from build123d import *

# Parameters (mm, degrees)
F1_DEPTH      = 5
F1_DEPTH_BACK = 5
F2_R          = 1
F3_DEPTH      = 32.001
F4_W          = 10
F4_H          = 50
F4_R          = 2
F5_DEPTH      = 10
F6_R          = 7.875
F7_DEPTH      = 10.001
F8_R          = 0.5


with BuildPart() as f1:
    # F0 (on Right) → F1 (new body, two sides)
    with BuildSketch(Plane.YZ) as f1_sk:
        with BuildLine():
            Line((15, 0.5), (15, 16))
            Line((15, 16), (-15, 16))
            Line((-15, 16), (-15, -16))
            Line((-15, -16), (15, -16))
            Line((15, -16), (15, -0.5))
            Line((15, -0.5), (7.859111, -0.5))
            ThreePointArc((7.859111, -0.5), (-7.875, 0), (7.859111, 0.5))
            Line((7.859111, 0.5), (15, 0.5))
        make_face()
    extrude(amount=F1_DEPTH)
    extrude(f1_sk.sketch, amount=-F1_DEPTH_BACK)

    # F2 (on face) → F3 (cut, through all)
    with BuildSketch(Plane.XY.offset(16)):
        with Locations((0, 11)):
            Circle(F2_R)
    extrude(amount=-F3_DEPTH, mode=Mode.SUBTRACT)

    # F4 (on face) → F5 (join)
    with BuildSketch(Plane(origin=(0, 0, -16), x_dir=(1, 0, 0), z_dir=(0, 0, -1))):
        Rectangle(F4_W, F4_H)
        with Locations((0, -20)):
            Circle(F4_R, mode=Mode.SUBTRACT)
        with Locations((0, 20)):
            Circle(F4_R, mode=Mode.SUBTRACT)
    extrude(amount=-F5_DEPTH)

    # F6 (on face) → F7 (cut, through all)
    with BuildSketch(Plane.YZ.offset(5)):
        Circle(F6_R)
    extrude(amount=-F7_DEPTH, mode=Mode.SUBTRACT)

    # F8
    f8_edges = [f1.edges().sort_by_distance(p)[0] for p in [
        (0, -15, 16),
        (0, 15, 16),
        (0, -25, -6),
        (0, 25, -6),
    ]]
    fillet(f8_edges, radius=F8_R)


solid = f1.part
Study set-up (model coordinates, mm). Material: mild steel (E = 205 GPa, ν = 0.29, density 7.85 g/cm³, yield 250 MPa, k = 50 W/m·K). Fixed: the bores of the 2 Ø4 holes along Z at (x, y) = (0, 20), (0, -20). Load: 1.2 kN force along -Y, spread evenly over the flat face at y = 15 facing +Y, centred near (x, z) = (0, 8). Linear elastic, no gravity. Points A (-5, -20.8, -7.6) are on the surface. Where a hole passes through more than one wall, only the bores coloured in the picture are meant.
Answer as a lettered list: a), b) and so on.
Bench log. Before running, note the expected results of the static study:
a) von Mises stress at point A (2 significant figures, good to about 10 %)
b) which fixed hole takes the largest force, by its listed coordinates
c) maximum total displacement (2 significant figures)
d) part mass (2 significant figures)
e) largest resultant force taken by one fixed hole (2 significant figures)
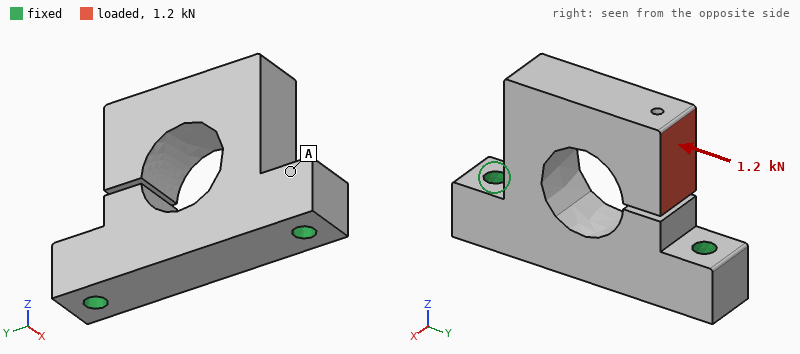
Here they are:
a) 19 MPa
b) (0, -20)
c) 71 µm
d) 73 g
e) 1.2 kN
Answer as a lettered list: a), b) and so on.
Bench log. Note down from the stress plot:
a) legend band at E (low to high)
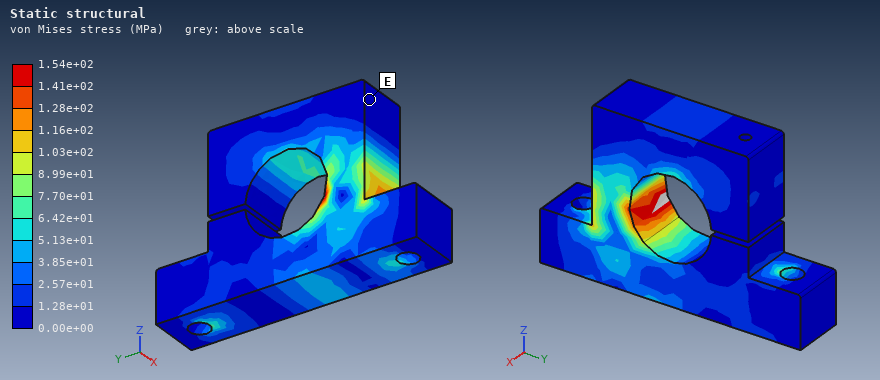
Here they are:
a) 0.00e+00 to 1.28e+01 MPa
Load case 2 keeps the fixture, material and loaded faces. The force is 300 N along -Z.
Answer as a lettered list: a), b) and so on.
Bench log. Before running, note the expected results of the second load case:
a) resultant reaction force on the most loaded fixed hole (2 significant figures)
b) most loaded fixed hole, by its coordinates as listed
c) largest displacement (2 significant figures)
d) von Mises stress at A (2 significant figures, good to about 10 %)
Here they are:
a) 260 N
b) (0, 20)
c) 67 µm
d) 6.2 MPa
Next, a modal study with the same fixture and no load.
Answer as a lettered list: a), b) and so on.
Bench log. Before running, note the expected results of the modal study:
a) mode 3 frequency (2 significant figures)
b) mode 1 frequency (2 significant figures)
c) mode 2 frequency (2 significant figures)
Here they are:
a) 7700 Hz
b) 3100 Hz
c) 3200 Hz
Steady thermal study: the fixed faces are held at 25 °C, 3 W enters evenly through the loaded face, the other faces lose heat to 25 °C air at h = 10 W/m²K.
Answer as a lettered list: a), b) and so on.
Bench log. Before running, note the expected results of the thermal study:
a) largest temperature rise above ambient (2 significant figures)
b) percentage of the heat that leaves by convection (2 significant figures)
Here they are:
a) 29 K
b) 12 %
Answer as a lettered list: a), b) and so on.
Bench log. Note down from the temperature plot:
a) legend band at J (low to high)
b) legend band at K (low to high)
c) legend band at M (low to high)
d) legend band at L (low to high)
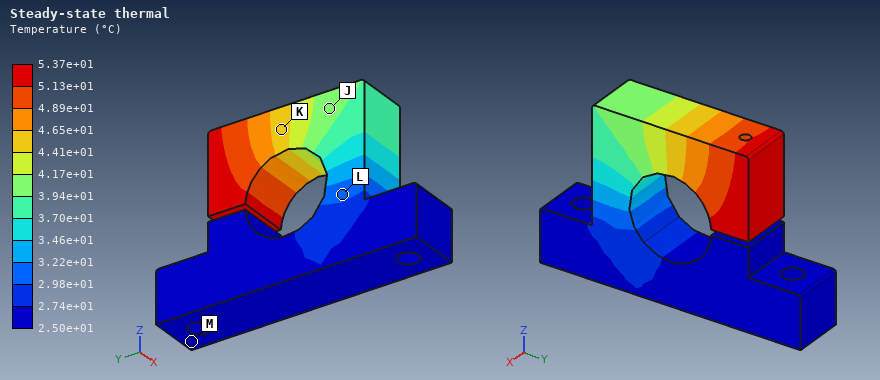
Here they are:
a) 3.94e+01 to 4.17e+01 °C
b) 4.41e+01 to 4.65e+01 °C
c) 2.50e+01 to 2.74e+01 °C
d) 2.98e+01 to 3.22e+01 °C
